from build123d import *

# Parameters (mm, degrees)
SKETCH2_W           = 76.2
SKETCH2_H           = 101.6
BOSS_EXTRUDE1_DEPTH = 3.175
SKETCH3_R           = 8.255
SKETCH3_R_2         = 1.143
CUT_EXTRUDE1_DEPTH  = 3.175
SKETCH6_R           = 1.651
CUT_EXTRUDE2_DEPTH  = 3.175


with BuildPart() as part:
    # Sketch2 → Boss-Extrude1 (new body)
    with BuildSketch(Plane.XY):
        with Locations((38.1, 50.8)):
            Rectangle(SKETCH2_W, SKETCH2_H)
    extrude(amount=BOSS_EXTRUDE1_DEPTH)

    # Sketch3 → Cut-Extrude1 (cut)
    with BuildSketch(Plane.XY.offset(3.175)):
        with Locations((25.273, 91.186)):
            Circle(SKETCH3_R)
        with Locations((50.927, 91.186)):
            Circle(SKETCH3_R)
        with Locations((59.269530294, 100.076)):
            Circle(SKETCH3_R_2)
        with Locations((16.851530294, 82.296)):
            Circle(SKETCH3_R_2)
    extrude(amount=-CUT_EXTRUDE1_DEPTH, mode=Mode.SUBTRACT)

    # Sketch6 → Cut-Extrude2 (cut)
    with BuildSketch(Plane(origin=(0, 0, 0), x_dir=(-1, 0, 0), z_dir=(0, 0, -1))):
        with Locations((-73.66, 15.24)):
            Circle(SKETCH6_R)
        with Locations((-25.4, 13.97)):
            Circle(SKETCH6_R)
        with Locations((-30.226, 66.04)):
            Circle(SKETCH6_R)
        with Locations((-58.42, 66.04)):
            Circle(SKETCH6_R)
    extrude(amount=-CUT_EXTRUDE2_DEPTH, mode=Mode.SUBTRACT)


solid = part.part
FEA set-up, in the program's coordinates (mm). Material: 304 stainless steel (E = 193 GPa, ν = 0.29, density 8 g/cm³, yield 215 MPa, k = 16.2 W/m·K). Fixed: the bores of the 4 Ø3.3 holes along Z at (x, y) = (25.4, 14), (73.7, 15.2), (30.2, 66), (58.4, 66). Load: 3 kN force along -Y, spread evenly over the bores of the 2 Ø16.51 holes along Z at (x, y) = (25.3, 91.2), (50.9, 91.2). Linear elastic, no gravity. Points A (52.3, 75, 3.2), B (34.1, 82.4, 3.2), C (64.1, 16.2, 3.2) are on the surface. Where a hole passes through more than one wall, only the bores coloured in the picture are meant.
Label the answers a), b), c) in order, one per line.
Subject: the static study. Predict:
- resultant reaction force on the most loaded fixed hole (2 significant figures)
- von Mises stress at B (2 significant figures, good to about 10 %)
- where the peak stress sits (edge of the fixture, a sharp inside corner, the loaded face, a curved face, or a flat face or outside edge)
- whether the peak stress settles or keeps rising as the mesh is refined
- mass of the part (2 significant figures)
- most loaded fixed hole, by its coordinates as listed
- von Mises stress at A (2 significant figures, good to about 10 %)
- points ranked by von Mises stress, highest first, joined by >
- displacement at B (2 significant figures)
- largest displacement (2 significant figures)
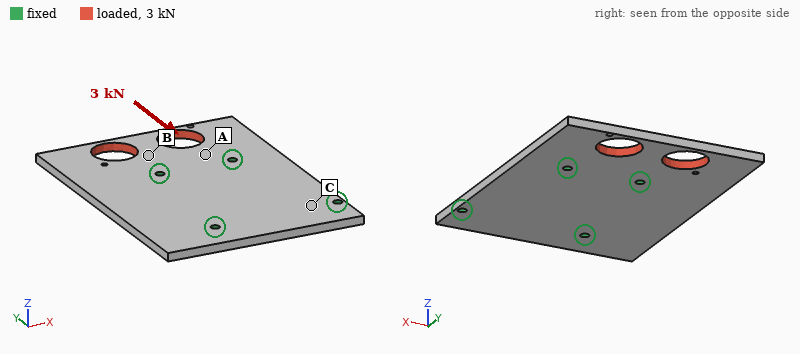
a) 1.5 kN
b) 27 MPa
c) edge of the fixture
d) keeps rising
e) 180 g
f) (30.2, 66)
g) 14 MPa
h) B > A > C
i) 2.5 µm
j) 8.2 µm
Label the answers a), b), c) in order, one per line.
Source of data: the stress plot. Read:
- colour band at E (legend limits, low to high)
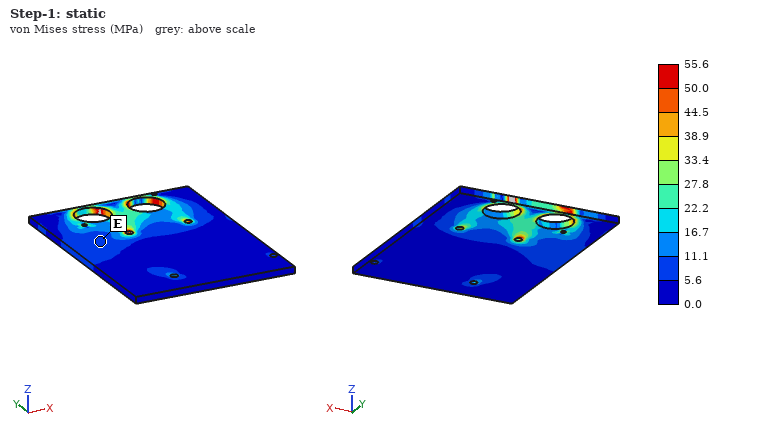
a) 5.6 to 11.1 MPa
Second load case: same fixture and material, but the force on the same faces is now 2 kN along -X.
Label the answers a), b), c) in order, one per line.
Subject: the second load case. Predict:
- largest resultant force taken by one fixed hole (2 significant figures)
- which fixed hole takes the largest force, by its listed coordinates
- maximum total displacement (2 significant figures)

a) 1.5 kN
b) (30.2, 66)
c) 13 µm
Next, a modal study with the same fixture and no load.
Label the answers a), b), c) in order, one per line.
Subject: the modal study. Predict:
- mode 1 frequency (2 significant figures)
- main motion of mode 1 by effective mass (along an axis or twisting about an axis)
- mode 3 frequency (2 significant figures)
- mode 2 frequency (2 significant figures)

a) 1700 Hz
b) along Z
c) 2700 Hz
d) 2200 Hz
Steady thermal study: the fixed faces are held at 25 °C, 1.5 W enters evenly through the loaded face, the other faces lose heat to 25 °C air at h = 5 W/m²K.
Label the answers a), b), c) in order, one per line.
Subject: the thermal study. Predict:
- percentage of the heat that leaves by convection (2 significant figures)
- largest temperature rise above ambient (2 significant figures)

a) 18 %
b) 18 K
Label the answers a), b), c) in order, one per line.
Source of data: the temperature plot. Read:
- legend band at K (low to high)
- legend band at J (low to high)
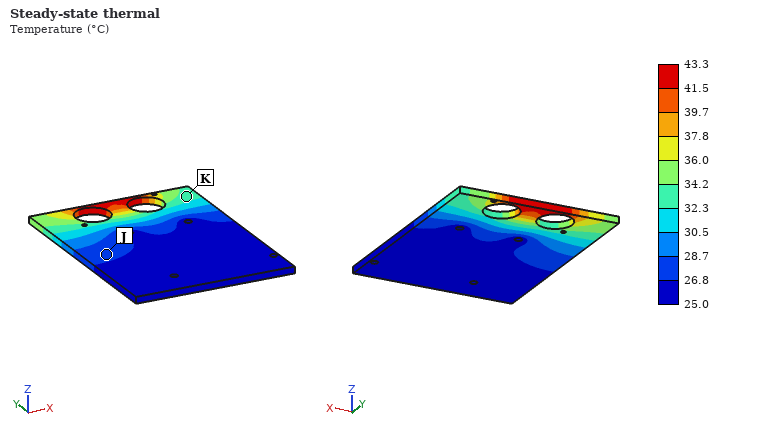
a) 32.3 to 34.2 °C
b) 26.8 to 28.7 °C
